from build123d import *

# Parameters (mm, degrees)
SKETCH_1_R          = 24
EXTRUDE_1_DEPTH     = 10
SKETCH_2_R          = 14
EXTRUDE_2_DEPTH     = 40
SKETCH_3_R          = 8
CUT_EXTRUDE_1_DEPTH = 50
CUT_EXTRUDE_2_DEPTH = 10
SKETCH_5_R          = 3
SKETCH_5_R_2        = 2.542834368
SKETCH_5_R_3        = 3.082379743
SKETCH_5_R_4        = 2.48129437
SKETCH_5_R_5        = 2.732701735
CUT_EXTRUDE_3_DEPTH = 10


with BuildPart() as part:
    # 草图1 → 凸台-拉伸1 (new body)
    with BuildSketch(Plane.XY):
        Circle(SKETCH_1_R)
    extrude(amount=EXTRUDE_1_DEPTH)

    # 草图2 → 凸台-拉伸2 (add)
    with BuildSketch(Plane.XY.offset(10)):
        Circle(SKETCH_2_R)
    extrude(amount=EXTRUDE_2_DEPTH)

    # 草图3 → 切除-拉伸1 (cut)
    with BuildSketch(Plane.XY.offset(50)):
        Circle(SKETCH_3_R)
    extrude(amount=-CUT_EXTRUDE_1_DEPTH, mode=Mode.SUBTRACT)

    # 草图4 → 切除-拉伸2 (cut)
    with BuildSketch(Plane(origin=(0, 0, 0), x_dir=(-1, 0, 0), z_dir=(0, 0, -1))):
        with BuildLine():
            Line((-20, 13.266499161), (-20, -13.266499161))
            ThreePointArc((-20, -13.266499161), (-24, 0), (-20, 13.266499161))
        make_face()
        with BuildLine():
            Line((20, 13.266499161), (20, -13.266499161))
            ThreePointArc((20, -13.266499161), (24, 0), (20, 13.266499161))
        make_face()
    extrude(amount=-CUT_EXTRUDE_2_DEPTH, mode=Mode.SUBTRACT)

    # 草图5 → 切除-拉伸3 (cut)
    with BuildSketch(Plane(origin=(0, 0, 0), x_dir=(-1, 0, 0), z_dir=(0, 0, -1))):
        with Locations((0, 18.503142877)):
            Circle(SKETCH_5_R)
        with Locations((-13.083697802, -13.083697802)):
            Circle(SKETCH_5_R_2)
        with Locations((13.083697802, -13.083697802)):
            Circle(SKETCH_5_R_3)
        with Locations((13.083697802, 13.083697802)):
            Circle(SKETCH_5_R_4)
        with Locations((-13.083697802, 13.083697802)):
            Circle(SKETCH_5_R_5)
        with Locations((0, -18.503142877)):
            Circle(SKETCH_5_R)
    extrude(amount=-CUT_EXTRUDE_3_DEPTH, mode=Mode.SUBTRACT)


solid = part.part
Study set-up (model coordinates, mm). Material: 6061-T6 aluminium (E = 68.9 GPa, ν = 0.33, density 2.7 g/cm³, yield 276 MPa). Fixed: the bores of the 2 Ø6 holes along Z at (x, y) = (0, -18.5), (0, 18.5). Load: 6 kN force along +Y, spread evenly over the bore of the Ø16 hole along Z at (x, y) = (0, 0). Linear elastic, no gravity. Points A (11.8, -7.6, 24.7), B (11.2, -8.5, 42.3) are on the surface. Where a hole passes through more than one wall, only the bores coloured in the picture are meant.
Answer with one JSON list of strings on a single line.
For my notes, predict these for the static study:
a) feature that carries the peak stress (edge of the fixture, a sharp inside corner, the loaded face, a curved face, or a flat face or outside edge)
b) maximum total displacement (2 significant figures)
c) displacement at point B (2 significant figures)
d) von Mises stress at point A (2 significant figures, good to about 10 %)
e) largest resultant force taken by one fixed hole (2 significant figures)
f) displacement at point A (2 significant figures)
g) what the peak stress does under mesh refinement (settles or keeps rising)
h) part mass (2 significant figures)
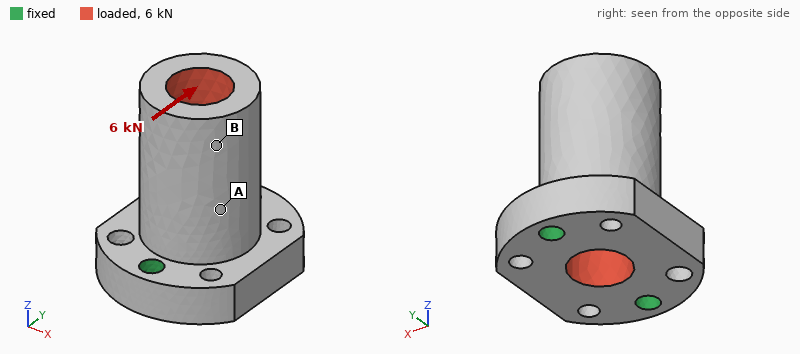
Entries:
["edge of the fixture", "61 µm", "49 µm", "19 MPa", "4.8 kN", "24 µm", "keeps rising", "80 g"]
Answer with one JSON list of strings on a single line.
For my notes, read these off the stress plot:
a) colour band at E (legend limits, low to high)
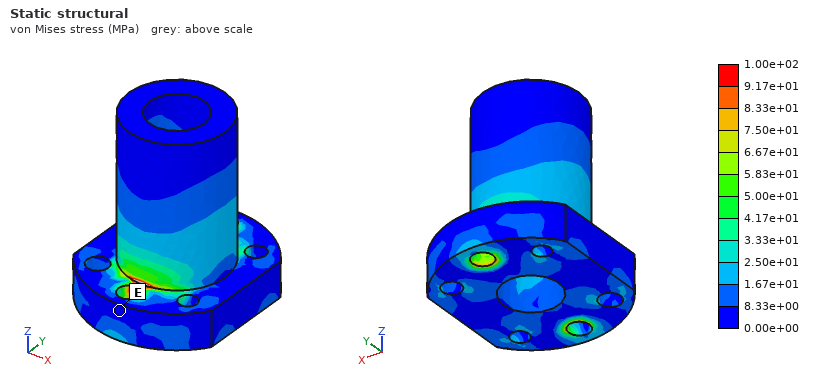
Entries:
["0.00e+00 to 8.33e+00 MPa"]
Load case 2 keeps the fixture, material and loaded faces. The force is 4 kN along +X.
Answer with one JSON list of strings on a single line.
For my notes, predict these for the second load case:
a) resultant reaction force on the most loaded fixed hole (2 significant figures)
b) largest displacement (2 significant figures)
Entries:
["2.0 kN", "0.12 mm"]
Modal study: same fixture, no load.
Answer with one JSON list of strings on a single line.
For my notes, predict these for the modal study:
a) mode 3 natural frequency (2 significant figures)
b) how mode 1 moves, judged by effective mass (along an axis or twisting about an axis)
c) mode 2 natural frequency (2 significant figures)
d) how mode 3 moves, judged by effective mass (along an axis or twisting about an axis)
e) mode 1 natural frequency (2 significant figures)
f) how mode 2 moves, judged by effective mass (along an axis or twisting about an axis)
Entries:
["15 kHz", "along X", "8000 Hz", "along Z", "4400 Hz", "along Y"]
